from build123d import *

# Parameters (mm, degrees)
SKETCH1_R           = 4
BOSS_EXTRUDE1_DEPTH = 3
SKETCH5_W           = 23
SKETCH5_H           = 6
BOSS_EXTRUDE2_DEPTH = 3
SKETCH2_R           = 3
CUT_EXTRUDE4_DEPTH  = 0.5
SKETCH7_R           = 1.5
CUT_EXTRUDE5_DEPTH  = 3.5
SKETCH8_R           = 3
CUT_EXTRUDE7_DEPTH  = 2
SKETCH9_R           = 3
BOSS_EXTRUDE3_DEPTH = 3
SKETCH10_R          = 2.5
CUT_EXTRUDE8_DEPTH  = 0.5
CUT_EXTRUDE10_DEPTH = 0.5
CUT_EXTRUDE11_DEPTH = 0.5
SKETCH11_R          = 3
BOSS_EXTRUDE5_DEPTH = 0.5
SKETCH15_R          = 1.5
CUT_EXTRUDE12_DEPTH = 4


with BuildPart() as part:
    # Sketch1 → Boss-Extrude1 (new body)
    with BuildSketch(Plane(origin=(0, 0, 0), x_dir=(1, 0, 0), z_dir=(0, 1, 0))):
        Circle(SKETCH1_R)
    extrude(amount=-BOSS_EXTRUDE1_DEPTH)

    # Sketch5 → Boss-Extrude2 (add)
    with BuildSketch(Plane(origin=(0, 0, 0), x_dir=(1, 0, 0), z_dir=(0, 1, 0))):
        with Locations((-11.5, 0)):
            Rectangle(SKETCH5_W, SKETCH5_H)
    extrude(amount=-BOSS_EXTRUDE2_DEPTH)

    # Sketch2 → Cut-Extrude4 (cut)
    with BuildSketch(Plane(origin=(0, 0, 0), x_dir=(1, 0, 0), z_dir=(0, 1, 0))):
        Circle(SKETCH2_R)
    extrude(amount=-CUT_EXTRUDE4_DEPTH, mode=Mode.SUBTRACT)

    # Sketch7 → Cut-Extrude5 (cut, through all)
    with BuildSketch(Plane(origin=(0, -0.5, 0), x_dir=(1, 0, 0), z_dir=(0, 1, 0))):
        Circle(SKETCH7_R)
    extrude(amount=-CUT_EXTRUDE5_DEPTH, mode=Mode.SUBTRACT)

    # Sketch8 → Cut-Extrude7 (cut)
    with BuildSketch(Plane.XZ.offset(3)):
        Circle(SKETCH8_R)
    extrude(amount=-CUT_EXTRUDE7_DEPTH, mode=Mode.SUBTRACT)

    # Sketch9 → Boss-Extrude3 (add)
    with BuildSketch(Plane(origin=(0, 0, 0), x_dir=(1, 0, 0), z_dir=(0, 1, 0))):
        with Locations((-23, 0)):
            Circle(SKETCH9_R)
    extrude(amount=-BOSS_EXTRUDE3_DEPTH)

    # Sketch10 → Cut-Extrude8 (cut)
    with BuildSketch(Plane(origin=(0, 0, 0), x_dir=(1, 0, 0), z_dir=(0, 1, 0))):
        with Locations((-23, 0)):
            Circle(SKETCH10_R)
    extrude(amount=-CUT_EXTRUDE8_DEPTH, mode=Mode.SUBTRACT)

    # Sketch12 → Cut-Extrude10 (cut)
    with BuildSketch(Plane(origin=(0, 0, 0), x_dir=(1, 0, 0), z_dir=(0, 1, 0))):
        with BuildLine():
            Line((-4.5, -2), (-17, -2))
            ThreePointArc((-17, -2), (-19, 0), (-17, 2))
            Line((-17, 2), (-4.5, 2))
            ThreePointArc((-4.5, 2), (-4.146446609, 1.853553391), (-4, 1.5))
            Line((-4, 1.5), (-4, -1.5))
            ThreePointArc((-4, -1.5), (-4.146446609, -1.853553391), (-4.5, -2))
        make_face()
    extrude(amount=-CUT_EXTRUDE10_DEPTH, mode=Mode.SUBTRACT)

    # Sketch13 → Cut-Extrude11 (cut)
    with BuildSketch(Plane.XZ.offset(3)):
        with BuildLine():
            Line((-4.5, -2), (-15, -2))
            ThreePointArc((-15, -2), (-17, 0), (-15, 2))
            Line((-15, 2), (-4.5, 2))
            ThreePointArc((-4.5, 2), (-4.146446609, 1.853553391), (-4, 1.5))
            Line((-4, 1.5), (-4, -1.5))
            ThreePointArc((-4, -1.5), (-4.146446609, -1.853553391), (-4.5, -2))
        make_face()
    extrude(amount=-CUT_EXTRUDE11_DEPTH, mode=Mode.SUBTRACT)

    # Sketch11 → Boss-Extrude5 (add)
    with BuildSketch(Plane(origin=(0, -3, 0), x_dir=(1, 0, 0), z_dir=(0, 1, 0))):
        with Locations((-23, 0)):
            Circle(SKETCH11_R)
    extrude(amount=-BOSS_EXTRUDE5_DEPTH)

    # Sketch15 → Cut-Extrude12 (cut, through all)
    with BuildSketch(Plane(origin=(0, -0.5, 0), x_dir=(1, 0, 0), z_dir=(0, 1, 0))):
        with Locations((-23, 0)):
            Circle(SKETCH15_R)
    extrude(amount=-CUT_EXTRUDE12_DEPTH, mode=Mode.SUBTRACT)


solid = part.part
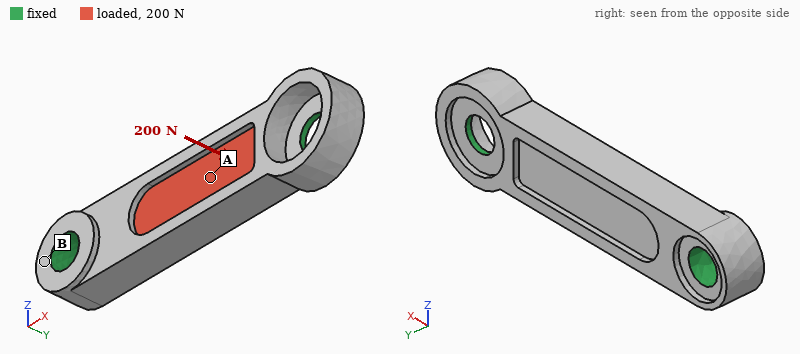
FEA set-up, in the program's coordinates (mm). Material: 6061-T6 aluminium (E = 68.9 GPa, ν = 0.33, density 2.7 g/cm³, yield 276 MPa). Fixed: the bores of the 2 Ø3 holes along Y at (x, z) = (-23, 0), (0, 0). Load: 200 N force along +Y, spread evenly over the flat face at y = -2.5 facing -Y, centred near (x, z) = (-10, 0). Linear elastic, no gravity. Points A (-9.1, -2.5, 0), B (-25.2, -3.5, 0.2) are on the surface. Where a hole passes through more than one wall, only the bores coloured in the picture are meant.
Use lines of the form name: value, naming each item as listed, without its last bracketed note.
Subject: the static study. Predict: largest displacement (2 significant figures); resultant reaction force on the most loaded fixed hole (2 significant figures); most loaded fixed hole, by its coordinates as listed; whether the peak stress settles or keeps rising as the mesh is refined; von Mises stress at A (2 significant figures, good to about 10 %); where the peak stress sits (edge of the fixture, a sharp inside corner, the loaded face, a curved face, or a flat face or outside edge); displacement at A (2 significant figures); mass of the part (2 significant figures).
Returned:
largest displacement: 25 µm
resultant reaction force on the most loaded fixed hole: 130 N
most loaded fixed hole, by its coordinates as listed: (-23, 0)
whether the peak stress settles or keeps rising as the mesh is refined: keeps rising
von Mises stress at A: 48 MPa
where the peak stress sits: edge of the fixture
displacement at A: 24 µm
mass of the part: 1.1 g
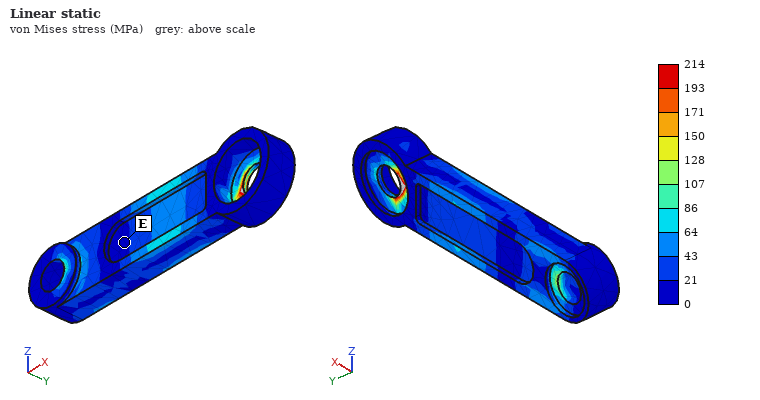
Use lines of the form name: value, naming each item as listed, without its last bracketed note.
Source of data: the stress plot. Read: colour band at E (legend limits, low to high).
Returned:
colour band at E: 0 to 21 MPa
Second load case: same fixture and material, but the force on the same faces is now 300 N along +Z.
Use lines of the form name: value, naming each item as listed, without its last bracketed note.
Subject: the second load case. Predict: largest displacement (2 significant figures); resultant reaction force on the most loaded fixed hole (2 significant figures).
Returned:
largest displacement: 21 µm
resultant reaction force on the most loaded fixed hole: 160 N
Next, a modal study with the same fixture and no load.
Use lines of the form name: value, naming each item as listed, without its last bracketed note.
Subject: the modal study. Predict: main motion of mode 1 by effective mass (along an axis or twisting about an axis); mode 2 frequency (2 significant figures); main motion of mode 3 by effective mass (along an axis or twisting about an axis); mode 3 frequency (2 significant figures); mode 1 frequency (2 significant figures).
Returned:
main motion of mode 1 by effective mass: along Y
mode 2 frequency: 29 kHz
main motion of mode 3 by effective mass: along Z
mode 3 frequency: 39 kHz
mode 1 frequency: 21 kHz
